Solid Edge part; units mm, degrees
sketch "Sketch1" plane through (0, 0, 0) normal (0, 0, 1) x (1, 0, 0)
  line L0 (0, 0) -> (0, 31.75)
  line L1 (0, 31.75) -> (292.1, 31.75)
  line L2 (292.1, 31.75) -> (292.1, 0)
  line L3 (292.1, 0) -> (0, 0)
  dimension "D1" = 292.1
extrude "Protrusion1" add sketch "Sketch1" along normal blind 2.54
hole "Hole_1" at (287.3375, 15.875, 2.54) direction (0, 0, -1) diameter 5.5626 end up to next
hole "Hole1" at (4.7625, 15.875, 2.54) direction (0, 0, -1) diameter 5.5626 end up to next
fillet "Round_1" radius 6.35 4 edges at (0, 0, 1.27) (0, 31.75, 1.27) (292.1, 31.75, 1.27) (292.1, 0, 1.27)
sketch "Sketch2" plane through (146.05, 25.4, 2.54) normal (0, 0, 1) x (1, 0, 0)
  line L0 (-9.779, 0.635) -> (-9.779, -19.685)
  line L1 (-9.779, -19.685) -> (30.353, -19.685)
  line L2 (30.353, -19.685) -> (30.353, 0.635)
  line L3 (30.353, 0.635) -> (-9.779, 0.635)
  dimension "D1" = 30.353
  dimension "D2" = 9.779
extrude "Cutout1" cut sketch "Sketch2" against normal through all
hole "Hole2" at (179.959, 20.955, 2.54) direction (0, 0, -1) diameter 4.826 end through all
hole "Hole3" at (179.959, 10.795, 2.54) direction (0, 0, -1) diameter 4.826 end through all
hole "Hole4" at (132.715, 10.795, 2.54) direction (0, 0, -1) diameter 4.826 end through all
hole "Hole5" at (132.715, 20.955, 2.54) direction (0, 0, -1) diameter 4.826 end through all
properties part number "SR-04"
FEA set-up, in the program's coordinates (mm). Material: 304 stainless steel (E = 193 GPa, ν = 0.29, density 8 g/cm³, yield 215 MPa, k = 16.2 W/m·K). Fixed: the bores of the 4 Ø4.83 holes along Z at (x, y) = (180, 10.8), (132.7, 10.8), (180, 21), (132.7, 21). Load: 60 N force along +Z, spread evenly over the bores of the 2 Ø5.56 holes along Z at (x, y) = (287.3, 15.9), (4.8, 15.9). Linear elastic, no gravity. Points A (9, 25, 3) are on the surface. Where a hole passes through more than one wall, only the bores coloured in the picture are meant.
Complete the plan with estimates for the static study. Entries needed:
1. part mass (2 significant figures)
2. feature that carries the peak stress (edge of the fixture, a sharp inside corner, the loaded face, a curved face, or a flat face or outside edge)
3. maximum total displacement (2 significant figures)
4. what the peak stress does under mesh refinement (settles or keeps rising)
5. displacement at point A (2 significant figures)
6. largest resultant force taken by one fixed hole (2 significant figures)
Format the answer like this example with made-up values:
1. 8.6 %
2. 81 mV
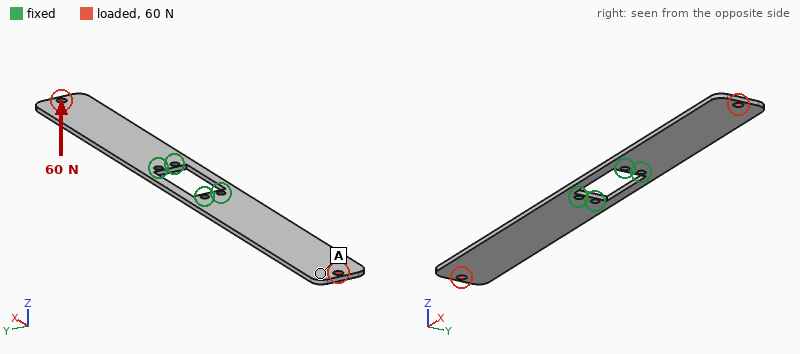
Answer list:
1. 170 g
2. edge of the fixture
3. 2.5 mm
4. keeps rising
5. 2.3 mm
6. 15 N
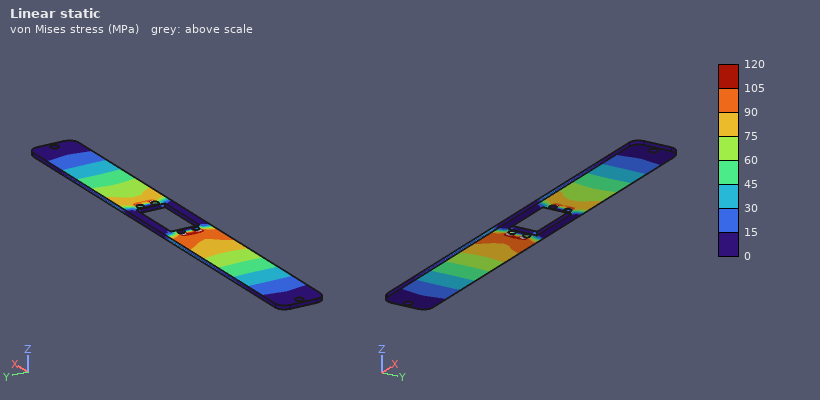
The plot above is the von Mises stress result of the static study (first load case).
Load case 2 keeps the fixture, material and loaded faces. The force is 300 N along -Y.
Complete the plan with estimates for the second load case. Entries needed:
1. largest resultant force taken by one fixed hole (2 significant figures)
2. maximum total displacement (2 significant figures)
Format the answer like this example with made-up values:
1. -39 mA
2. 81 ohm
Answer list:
1. 890 N
2. 0.11 mm
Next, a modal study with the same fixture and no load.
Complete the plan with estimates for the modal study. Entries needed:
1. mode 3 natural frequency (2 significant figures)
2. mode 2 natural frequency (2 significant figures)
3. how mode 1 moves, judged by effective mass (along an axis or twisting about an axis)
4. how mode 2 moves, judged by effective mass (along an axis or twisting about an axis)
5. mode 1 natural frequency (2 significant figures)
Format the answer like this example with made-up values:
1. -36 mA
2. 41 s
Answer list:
1. 750 Hz
2. 170 Hz
3. along Z
4. along Z
5. 120 Hz
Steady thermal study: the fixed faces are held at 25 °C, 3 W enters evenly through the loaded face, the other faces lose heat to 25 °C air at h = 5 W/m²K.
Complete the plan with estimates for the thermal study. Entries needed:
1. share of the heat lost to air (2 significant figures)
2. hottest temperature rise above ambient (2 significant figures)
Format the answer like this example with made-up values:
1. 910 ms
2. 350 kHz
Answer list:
1. 73 %
2. 74 K
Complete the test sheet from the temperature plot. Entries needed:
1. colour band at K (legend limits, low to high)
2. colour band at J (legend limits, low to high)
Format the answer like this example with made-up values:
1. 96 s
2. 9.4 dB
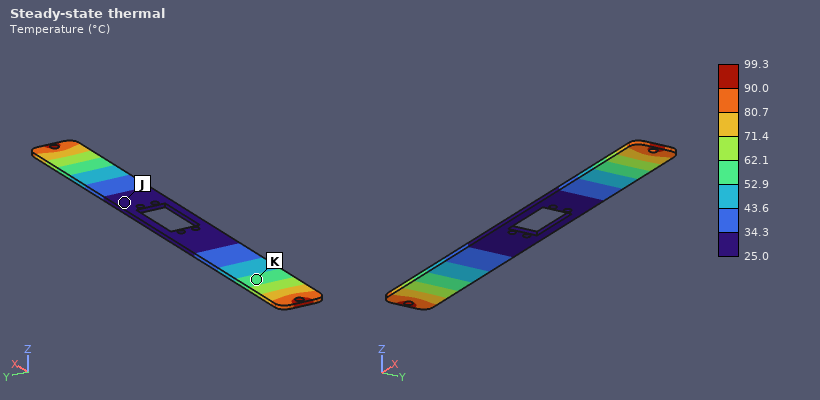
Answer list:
1. 52.9 to 62.1 °C
2. 25.0 to 34.3 °C
